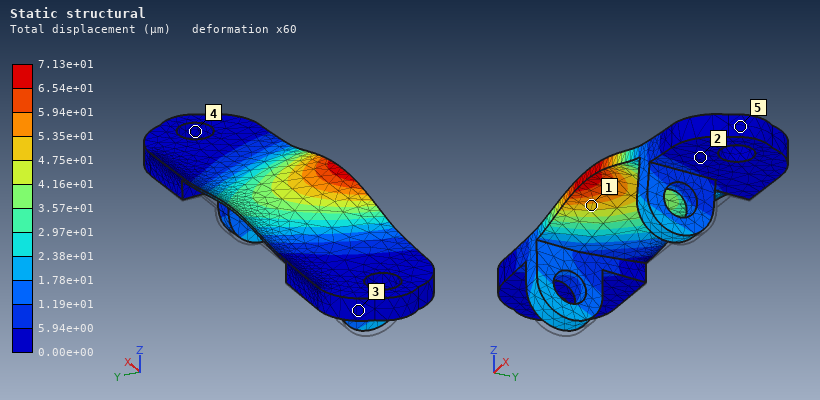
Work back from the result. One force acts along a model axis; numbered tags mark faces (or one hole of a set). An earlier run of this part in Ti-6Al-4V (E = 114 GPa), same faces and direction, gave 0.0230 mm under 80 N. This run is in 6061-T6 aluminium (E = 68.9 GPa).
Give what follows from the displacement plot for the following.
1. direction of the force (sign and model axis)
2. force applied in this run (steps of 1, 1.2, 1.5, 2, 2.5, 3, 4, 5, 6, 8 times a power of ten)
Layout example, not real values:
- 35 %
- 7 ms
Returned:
- +Z
- 150 N
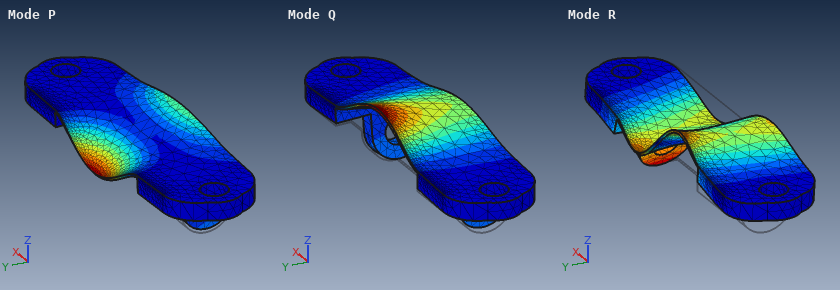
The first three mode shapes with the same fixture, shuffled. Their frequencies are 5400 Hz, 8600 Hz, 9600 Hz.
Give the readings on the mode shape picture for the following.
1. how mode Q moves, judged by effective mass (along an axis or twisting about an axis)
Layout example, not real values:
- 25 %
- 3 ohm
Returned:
- along Z
